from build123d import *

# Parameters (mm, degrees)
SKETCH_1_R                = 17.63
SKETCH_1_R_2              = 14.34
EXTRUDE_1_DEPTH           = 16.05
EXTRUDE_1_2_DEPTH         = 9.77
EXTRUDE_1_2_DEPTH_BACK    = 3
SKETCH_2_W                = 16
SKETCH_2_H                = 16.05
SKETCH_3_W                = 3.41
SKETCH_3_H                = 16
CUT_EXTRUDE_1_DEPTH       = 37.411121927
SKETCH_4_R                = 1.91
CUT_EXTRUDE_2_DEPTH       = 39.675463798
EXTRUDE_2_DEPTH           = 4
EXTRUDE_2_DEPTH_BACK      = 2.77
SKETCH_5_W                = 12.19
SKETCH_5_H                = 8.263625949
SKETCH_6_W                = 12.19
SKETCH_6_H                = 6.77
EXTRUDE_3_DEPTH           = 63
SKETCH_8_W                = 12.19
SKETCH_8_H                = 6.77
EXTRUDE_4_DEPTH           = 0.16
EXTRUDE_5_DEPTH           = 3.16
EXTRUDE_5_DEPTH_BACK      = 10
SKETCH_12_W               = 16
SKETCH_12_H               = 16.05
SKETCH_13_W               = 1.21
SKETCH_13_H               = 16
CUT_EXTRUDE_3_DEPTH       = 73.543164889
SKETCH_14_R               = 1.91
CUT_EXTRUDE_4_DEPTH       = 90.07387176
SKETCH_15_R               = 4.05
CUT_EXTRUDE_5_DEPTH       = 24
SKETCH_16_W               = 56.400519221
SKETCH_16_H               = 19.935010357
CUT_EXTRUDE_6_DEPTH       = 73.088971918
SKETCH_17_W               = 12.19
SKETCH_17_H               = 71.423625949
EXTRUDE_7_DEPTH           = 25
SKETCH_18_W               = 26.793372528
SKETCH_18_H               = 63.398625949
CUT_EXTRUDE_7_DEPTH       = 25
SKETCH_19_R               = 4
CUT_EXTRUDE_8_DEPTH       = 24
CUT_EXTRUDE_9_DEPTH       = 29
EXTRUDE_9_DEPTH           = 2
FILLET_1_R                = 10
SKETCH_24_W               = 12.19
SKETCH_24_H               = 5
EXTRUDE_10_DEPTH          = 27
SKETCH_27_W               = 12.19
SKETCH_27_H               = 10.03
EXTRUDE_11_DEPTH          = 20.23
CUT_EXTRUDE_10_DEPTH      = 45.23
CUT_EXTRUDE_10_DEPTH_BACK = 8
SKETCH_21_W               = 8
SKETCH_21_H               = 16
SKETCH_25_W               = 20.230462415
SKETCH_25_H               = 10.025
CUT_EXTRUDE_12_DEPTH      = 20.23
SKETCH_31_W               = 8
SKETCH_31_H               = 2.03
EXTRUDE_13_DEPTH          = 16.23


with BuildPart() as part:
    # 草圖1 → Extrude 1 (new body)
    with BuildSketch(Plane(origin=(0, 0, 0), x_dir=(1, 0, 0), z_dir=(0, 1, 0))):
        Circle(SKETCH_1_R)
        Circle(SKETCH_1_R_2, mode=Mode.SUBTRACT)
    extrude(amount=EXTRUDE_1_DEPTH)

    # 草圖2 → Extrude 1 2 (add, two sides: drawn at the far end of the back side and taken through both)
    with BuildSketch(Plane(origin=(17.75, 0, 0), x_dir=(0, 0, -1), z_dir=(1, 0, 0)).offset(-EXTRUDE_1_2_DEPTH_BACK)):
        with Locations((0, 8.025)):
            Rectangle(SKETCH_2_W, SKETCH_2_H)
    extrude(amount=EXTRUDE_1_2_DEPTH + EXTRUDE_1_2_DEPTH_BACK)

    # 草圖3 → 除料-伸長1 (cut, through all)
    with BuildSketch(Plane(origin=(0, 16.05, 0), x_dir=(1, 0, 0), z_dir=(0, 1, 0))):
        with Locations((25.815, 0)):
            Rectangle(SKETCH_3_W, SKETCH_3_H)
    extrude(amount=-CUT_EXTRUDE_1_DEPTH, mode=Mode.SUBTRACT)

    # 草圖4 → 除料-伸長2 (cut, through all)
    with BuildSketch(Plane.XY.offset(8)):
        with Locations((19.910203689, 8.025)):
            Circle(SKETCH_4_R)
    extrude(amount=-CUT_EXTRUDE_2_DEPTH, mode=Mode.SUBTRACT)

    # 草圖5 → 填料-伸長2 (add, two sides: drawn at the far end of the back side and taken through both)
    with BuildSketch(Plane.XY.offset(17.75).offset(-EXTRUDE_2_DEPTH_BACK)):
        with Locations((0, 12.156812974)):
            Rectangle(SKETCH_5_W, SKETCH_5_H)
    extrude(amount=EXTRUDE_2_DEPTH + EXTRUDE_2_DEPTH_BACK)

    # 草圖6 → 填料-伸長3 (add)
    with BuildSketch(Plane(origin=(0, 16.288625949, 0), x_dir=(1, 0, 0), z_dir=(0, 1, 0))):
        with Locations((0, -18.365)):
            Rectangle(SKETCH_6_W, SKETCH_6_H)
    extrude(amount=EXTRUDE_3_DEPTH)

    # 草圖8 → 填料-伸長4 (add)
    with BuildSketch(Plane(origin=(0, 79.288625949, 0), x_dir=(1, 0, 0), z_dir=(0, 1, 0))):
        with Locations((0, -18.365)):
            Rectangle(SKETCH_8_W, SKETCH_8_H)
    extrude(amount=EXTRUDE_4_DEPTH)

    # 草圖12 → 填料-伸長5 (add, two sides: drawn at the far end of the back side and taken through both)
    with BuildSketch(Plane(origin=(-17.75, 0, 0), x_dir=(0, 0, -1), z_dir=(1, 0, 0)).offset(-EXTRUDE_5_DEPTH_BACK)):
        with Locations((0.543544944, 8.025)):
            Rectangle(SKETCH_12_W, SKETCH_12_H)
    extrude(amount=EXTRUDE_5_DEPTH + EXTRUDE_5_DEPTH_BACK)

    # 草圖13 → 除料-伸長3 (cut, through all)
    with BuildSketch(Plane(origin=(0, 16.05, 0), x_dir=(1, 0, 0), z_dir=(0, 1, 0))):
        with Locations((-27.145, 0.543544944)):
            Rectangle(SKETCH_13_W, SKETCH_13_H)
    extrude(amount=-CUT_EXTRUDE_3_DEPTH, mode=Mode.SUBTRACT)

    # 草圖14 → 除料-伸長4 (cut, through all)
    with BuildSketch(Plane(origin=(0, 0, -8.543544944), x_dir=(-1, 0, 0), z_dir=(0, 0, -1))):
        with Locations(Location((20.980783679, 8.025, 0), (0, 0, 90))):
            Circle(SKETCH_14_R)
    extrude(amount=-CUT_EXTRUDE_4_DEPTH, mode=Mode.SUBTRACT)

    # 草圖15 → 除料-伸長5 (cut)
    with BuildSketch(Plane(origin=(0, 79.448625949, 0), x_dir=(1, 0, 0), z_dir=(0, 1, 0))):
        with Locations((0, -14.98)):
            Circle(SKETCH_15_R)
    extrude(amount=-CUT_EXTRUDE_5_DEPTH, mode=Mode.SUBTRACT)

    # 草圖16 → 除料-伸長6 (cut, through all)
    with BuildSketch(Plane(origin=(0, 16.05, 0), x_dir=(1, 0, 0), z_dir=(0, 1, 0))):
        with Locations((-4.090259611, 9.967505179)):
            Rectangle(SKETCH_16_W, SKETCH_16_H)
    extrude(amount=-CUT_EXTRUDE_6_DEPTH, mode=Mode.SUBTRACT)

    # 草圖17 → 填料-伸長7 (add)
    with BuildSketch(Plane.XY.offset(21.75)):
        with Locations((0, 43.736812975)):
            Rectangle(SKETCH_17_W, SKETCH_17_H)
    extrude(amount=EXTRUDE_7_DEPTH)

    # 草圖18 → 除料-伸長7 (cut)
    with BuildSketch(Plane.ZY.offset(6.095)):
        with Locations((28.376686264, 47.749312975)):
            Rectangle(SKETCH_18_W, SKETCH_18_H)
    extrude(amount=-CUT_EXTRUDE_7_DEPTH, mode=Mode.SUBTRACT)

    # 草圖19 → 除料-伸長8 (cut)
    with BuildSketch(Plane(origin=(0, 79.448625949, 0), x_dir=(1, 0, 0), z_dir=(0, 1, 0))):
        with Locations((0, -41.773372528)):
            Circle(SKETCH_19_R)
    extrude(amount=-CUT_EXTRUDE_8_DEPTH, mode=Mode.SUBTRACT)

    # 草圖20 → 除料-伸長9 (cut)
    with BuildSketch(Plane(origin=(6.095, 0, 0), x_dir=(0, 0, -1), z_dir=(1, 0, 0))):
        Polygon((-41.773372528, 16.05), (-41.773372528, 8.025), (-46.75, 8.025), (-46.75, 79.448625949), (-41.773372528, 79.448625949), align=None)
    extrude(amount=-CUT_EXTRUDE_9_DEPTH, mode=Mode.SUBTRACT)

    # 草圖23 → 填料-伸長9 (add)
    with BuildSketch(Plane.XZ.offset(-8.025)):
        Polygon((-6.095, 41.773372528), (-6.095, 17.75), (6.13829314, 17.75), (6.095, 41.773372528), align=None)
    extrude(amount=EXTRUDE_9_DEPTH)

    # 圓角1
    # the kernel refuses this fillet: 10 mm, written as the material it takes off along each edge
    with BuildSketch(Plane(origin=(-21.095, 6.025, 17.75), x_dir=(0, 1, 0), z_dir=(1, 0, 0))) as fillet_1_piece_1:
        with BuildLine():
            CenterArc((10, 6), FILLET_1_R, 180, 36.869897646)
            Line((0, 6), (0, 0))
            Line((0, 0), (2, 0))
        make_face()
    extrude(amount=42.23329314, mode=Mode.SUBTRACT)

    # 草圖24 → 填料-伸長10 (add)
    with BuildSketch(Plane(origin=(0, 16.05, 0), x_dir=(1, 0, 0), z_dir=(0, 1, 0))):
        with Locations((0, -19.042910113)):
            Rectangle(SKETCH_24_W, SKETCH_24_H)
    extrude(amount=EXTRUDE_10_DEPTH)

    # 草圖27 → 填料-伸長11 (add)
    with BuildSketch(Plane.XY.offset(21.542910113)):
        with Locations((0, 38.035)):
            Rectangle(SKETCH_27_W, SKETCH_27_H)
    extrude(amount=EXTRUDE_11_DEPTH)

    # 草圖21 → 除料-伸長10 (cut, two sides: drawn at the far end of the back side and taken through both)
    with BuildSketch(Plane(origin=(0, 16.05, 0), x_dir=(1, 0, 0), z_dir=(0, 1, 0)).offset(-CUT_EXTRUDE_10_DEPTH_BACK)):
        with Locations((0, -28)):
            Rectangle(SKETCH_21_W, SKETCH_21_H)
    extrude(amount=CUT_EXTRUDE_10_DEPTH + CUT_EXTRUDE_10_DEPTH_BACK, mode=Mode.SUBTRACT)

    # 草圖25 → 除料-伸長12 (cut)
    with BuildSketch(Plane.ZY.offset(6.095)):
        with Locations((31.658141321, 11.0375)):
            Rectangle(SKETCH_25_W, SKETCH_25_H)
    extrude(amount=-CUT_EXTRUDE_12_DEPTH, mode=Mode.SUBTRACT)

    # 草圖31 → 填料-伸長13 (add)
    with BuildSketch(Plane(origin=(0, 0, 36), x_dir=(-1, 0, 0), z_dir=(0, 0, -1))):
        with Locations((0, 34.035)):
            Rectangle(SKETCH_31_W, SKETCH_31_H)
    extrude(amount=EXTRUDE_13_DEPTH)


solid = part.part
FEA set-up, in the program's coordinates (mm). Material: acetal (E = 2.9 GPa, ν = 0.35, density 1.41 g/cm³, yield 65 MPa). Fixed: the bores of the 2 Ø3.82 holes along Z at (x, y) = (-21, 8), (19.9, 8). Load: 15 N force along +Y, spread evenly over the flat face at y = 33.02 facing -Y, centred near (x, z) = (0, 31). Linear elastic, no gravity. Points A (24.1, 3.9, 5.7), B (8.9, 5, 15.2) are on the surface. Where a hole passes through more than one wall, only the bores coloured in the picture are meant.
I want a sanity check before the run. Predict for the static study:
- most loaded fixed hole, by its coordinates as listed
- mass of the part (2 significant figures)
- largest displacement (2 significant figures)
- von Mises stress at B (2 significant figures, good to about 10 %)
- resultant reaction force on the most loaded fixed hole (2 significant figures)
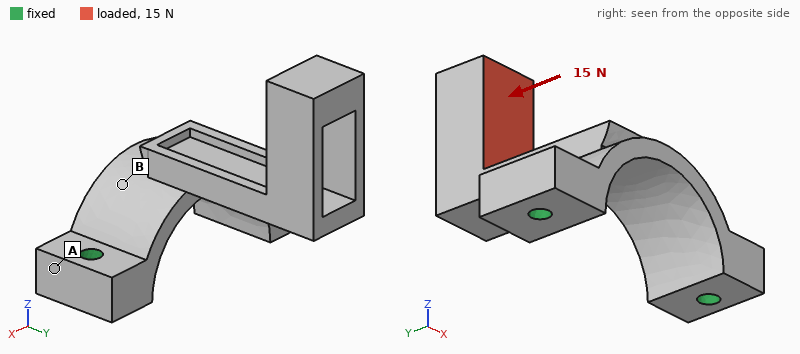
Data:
(19.9, 8)
11 g
0.71 mm
1.4 MPa
8.2 N
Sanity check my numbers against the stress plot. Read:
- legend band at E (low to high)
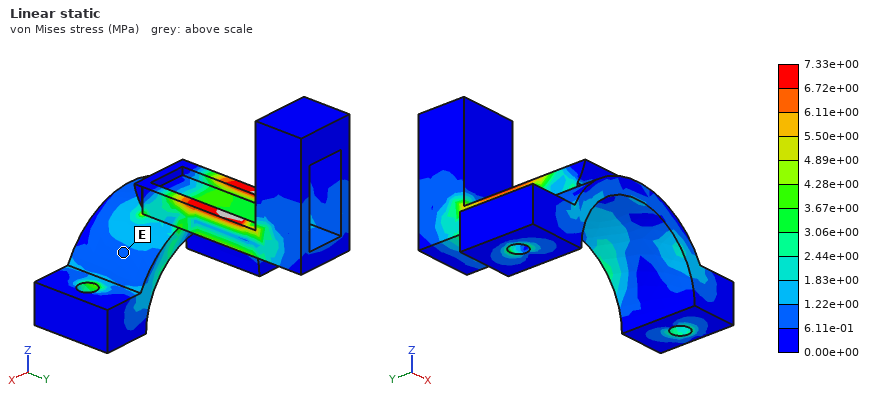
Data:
6.11e-01 to 1.22e+00 MPa
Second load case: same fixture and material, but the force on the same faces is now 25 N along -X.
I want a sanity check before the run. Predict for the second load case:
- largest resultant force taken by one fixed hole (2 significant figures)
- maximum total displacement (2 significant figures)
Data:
31 N
0.80 mm
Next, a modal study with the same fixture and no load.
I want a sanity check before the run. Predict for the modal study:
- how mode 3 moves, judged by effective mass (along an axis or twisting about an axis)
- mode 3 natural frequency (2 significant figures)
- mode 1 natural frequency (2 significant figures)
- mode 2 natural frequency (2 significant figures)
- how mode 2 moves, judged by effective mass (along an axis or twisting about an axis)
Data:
along Z
1600 Hz
400 Hz
620 Hz
along X
